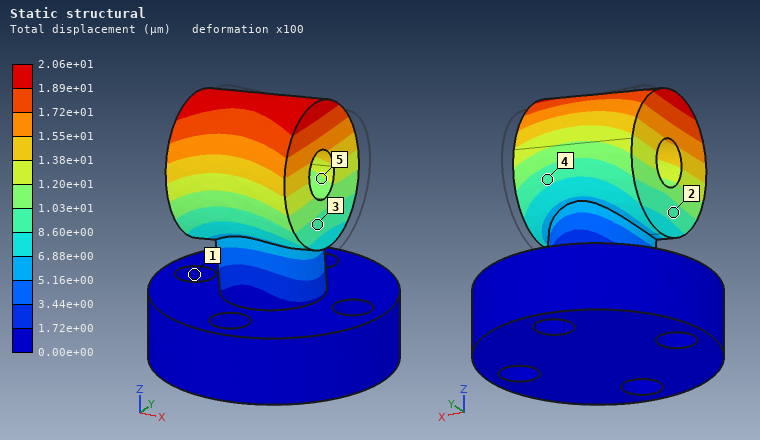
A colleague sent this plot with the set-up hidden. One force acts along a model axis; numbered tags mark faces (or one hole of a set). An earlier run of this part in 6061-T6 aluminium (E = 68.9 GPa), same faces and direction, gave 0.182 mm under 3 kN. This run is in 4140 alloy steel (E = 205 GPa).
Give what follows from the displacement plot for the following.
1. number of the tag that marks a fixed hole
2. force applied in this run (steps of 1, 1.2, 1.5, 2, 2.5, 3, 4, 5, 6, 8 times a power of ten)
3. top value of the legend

1
1 kN
2.06e+01 µm
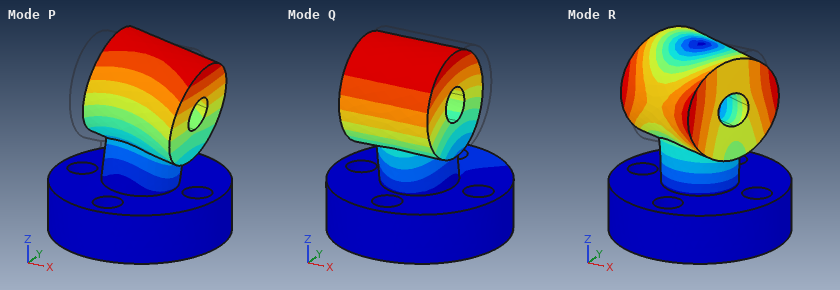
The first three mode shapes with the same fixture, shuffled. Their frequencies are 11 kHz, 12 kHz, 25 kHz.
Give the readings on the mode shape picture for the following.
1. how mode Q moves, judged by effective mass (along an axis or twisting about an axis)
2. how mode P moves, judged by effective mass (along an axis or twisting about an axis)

along Y
along X
